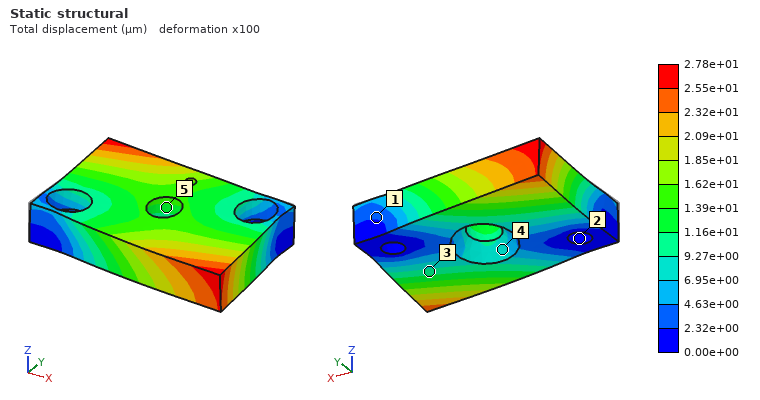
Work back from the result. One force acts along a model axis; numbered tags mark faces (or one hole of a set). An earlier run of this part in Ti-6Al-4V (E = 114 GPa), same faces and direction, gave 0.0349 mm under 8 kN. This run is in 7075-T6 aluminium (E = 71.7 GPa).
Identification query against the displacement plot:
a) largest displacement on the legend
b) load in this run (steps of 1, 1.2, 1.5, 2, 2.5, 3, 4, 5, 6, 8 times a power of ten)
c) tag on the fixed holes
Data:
2.78e+01 µm
4 kN
2
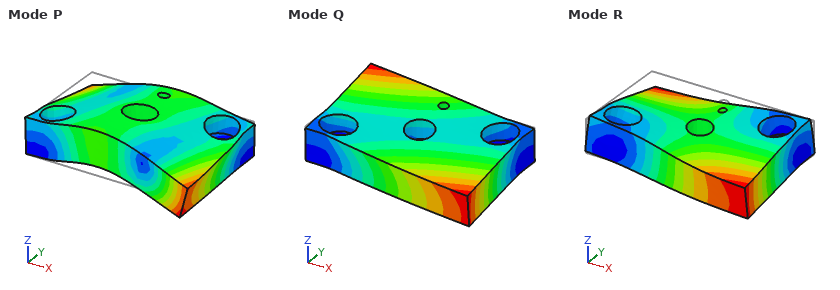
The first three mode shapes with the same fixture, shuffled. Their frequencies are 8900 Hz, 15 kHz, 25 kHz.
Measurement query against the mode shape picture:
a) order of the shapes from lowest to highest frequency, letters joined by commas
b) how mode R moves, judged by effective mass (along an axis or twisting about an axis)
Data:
Q, R, P
along Z
